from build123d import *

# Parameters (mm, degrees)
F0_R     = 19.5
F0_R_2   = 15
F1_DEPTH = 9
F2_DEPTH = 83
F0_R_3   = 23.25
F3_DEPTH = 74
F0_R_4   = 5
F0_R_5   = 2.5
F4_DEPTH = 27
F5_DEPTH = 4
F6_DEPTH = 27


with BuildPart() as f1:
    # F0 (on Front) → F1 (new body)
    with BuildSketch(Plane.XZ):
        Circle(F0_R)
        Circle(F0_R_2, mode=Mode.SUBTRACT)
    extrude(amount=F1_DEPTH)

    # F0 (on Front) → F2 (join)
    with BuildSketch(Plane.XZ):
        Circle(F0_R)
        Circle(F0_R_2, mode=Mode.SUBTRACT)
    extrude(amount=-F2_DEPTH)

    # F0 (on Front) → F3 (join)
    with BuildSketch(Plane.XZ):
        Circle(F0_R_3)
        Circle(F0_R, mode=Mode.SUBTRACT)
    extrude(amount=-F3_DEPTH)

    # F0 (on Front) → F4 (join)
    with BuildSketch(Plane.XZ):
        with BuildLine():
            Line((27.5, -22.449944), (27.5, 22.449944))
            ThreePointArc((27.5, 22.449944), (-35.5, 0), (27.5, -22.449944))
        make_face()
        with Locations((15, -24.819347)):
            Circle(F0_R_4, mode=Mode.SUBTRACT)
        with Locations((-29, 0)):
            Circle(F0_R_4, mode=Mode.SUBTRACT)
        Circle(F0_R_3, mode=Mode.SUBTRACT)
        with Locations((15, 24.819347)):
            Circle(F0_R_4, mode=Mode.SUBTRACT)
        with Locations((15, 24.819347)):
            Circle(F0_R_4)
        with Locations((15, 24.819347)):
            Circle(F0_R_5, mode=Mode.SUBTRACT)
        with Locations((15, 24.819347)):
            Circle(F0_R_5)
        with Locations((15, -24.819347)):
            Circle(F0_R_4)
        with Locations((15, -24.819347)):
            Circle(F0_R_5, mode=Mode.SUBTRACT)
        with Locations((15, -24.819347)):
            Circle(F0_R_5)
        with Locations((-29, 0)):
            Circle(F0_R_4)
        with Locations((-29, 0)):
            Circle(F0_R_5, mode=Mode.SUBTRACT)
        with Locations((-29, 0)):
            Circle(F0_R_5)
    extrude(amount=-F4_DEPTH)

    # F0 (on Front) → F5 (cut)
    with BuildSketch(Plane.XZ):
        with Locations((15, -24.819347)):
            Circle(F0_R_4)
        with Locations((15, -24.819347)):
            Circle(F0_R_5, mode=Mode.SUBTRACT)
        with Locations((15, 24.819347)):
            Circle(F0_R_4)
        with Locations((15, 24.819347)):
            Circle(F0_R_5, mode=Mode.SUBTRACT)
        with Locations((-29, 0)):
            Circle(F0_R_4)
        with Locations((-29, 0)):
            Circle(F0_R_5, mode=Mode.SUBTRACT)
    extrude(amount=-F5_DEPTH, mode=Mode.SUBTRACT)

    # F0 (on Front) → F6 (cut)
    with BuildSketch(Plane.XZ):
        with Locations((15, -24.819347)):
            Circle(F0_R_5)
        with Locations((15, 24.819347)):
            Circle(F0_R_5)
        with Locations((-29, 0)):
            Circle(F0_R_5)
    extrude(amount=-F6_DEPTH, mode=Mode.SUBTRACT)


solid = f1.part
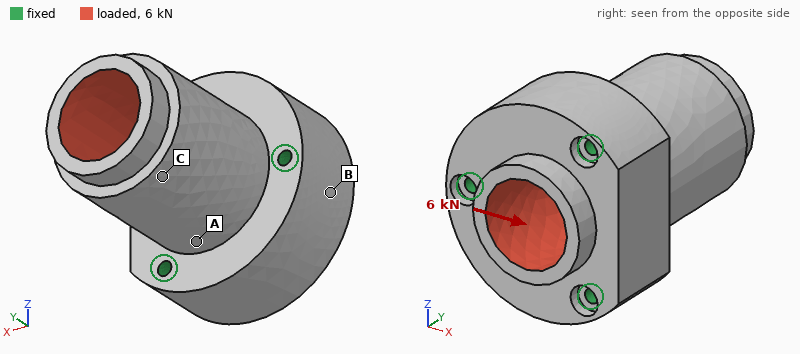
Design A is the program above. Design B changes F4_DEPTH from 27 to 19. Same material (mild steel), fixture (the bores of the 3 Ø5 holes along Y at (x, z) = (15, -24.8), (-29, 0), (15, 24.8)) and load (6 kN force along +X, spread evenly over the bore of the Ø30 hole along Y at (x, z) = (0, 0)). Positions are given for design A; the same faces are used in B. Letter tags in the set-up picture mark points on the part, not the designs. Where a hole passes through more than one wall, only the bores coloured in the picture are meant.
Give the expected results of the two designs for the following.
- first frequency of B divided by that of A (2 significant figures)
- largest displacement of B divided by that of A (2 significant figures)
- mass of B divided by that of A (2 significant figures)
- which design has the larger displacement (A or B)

0.77
1.6
0.88
B
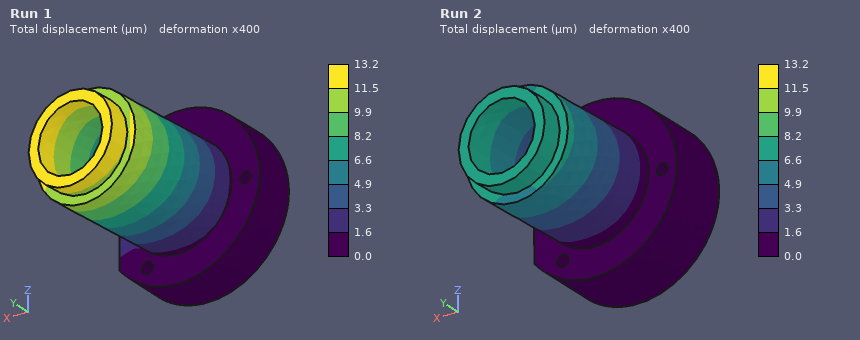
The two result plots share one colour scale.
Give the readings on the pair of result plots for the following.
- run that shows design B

Run 1
